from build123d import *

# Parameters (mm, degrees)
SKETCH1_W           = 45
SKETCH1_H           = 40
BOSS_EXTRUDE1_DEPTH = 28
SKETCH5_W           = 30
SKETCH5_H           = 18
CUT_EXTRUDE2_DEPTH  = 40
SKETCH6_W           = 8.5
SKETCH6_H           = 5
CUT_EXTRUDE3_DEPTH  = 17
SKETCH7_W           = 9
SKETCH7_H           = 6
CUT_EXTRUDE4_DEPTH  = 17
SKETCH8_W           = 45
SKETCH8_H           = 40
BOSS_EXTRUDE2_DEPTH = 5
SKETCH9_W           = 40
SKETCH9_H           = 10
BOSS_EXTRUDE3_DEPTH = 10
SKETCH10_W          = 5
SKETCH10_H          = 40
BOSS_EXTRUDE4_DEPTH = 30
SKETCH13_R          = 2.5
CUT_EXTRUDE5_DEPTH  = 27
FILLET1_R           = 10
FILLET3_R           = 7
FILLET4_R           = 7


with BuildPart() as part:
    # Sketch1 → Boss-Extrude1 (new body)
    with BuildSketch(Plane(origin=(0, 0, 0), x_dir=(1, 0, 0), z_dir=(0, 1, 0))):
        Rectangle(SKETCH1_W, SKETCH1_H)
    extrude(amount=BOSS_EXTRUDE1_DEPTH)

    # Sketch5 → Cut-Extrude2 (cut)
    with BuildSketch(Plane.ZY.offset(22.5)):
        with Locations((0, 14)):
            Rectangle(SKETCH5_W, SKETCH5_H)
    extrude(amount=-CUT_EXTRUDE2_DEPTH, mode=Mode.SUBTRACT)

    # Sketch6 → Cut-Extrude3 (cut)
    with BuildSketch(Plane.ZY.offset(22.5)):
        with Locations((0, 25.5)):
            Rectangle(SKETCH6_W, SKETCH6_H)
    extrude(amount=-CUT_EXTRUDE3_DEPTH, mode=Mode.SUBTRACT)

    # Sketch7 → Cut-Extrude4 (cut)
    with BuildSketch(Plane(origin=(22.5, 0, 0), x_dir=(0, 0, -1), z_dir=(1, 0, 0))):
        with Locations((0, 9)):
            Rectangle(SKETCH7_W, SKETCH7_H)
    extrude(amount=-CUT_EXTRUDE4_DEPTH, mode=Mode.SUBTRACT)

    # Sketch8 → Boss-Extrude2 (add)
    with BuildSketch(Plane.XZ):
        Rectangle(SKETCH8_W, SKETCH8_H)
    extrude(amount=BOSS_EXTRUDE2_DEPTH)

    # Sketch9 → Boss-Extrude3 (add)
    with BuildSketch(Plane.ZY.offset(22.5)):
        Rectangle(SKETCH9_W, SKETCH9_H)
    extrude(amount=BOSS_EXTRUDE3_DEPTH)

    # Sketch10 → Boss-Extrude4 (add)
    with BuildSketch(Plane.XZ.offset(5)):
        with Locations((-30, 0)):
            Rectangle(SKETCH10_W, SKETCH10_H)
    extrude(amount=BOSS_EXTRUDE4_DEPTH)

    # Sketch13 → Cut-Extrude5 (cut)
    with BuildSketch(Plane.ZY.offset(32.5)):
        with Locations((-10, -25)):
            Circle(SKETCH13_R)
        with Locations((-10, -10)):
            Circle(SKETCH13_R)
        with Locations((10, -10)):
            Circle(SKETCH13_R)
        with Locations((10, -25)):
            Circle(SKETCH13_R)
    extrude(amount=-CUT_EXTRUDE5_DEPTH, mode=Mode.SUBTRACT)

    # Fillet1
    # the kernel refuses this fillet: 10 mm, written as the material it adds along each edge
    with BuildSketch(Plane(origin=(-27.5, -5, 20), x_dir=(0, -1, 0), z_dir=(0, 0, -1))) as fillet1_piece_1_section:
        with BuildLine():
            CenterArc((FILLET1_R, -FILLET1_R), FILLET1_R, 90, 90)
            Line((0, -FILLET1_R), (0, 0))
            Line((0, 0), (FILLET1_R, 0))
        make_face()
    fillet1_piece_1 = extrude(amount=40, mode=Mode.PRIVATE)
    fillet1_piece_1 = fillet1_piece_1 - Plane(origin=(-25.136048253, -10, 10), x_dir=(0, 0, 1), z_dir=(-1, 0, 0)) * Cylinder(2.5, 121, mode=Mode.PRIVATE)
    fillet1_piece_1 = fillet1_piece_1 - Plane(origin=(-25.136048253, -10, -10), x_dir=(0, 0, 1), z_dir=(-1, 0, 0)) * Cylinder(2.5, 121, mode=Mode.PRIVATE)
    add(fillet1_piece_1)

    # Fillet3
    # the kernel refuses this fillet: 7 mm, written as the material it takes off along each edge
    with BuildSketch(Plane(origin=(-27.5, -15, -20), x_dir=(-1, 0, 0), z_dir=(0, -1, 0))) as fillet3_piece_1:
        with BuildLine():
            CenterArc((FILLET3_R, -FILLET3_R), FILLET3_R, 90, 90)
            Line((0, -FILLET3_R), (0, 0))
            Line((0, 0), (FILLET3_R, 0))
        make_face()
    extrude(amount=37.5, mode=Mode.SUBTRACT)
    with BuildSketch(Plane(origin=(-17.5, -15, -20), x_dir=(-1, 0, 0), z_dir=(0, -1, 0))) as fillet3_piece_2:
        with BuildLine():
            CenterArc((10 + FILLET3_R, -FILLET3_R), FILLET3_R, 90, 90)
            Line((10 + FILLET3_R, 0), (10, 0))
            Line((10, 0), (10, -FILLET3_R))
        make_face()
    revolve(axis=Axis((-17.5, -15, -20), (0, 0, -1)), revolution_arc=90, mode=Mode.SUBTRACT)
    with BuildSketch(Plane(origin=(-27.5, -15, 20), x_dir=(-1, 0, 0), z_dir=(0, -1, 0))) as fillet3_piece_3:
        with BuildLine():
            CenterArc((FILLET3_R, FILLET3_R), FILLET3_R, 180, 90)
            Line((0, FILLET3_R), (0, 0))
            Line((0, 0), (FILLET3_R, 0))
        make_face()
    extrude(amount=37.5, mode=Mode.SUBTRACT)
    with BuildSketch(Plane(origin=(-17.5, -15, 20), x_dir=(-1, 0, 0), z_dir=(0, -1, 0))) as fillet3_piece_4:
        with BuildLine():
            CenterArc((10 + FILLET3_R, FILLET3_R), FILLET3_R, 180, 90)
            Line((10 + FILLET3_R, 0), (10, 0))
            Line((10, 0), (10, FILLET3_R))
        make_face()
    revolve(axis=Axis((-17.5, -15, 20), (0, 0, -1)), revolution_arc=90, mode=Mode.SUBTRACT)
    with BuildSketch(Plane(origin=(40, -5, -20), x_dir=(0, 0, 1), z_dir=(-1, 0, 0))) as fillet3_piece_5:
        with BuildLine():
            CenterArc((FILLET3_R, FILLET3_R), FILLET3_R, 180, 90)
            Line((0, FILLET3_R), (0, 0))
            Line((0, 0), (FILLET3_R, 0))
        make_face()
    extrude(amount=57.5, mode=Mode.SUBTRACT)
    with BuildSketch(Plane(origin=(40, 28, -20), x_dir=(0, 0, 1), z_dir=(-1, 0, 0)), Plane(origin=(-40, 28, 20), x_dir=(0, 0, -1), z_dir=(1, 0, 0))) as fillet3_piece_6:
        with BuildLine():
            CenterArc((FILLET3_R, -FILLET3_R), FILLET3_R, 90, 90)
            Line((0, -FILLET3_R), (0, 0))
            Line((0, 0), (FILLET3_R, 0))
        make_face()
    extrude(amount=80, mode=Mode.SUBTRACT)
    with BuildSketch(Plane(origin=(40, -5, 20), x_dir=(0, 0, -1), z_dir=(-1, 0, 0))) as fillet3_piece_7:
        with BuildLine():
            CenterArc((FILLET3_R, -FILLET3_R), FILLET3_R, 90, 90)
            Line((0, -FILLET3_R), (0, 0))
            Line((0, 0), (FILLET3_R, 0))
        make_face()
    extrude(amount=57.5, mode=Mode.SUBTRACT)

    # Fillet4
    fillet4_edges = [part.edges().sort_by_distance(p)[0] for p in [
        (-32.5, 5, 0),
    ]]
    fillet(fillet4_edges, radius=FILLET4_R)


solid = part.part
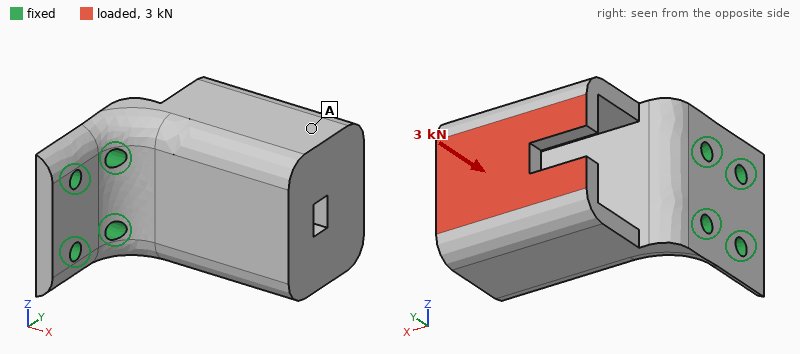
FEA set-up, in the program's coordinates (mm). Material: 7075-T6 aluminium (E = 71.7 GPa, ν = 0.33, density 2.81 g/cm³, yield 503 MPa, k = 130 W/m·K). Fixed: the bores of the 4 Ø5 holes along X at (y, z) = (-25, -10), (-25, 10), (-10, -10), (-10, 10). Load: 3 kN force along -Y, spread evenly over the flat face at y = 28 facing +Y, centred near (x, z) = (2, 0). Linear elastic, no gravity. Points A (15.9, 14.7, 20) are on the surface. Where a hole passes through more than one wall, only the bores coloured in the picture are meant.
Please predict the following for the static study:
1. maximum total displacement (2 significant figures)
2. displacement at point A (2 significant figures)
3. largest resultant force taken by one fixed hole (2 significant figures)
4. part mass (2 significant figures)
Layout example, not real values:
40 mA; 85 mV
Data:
0.48 mm; 0.38 mm; 2.0 kN; 120 g
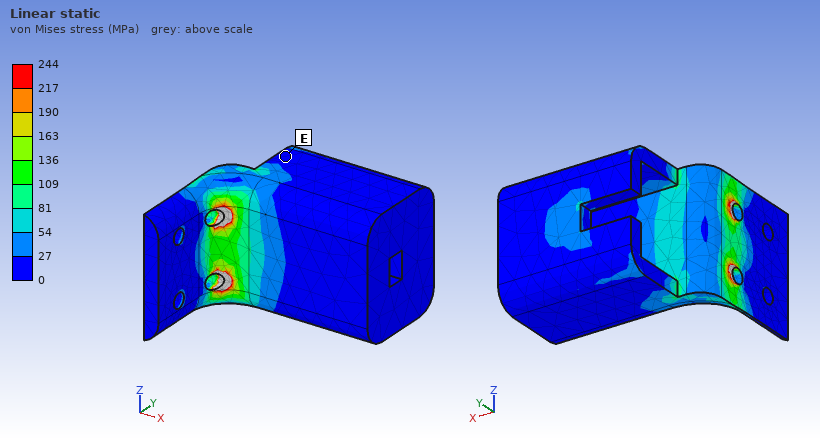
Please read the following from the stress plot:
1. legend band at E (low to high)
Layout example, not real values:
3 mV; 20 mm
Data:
0 to 27 MPa
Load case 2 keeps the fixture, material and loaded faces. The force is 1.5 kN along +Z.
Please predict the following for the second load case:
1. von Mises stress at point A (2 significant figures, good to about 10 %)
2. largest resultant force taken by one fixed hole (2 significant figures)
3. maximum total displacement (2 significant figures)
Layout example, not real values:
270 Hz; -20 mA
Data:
14 MPa; 2.9 kN; 0.11 mm
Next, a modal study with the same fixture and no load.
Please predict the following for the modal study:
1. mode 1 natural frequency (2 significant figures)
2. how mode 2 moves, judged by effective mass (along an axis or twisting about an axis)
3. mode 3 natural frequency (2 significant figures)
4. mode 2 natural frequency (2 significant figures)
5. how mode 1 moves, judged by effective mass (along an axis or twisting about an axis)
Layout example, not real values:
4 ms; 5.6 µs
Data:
1400 Hz; along Z; 4100 Hz; 3300 Hz; along Y
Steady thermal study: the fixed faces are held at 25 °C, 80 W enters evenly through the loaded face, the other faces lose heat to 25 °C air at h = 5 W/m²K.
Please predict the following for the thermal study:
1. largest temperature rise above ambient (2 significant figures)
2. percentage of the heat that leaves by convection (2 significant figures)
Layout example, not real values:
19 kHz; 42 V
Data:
80 K; 3.8 %
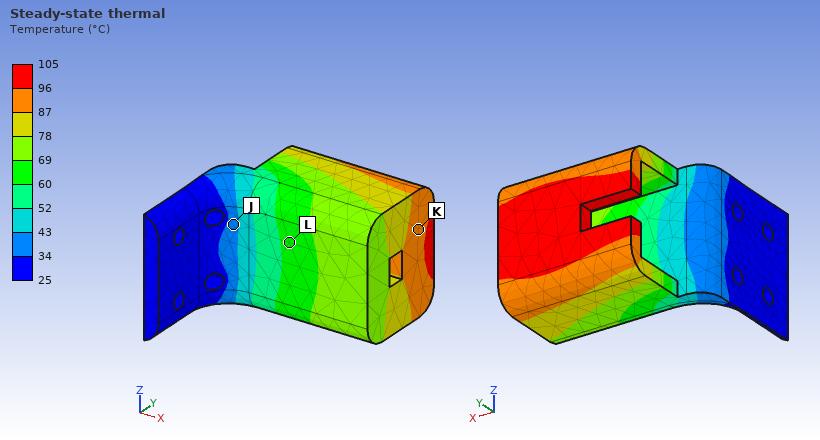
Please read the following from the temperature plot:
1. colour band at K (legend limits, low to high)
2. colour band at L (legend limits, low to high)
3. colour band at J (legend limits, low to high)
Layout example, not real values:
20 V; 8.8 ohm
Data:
87 to 96 °C; 60 to 69 °C; 34 to 43 °C
